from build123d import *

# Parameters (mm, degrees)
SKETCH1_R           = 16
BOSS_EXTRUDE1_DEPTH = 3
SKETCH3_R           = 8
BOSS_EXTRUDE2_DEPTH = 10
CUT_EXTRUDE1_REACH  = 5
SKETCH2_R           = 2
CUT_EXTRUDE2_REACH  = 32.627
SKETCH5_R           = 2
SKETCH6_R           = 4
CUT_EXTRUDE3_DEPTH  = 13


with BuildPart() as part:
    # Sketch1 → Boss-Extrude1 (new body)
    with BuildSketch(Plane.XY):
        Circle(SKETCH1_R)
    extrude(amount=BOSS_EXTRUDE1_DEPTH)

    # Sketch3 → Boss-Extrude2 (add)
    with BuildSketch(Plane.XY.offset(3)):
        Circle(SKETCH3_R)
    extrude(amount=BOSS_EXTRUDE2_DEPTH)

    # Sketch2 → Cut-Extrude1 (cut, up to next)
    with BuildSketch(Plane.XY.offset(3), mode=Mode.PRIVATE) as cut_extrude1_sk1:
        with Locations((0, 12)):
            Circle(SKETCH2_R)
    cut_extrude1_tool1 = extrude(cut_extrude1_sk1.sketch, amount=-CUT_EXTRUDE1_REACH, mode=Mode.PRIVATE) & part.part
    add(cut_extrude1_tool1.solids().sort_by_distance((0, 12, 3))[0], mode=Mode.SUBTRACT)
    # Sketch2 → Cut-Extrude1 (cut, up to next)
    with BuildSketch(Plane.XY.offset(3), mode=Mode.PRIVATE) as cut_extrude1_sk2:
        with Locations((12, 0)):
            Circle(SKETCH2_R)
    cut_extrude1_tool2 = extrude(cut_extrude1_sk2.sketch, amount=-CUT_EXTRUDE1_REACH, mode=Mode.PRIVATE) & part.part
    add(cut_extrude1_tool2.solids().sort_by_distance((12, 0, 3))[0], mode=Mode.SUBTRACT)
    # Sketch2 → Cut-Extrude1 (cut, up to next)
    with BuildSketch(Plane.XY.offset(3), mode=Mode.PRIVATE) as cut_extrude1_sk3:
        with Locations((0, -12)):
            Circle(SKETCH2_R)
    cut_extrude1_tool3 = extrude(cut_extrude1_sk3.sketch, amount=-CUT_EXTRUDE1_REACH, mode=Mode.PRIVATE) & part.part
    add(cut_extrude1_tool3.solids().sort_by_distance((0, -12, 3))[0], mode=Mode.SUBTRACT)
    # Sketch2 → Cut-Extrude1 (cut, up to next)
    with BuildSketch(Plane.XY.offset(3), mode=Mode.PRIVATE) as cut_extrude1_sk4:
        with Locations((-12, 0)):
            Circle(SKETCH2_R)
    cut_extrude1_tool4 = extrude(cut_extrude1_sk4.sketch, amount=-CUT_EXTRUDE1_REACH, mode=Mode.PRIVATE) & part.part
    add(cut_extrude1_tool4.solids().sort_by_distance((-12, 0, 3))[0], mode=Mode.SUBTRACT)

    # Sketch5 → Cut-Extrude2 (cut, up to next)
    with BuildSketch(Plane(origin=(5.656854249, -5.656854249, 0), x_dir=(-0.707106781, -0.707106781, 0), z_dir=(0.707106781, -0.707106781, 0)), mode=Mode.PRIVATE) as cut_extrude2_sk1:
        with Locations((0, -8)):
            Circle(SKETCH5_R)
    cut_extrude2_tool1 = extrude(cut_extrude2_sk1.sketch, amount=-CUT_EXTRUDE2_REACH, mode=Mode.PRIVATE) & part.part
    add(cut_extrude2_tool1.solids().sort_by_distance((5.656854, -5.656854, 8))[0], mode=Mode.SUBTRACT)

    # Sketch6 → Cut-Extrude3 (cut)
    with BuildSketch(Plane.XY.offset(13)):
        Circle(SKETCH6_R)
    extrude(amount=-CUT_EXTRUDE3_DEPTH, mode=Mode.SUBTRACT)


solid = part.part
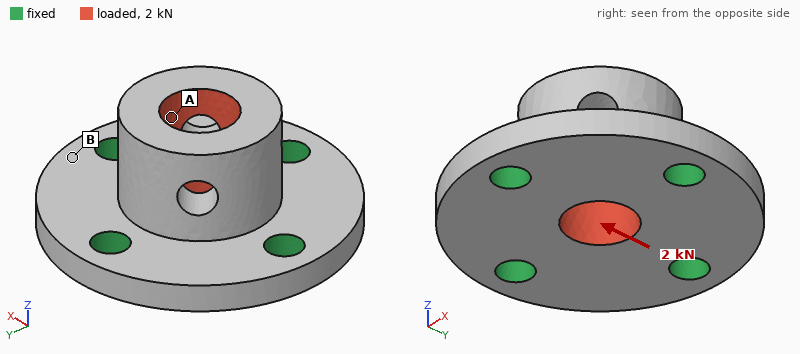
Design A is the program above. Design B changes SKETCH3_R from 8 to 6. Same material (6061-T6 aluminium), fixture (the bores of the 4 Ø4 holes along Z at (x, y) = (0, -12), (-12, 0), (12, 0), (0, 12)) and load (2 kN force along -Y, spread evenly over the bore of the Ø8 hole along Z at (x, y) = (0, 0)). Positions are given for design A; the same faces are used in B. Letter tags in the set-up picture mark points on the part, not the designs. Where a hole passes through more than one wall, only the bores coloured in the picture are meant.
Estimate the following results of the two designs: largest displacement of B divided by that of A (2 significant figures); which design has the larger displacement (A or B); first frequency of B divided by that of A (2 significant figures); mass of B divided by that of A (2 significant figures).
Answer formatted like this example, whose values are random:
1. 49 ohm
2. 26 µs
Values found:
1. 2.8
2. B
3. 0.93
4. 0.76
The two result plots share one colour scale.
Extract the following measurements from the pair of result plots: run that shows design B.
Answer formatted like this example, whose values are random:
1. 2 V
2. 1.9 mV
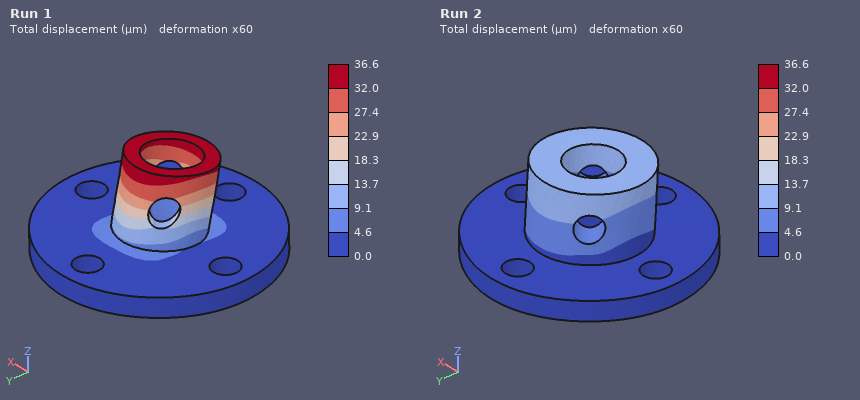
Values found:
1. Run 1
